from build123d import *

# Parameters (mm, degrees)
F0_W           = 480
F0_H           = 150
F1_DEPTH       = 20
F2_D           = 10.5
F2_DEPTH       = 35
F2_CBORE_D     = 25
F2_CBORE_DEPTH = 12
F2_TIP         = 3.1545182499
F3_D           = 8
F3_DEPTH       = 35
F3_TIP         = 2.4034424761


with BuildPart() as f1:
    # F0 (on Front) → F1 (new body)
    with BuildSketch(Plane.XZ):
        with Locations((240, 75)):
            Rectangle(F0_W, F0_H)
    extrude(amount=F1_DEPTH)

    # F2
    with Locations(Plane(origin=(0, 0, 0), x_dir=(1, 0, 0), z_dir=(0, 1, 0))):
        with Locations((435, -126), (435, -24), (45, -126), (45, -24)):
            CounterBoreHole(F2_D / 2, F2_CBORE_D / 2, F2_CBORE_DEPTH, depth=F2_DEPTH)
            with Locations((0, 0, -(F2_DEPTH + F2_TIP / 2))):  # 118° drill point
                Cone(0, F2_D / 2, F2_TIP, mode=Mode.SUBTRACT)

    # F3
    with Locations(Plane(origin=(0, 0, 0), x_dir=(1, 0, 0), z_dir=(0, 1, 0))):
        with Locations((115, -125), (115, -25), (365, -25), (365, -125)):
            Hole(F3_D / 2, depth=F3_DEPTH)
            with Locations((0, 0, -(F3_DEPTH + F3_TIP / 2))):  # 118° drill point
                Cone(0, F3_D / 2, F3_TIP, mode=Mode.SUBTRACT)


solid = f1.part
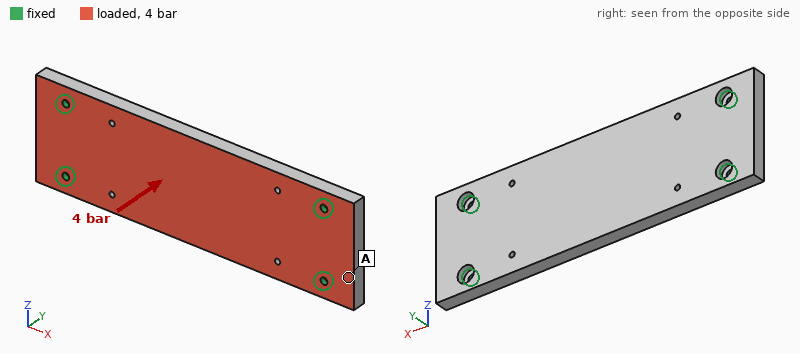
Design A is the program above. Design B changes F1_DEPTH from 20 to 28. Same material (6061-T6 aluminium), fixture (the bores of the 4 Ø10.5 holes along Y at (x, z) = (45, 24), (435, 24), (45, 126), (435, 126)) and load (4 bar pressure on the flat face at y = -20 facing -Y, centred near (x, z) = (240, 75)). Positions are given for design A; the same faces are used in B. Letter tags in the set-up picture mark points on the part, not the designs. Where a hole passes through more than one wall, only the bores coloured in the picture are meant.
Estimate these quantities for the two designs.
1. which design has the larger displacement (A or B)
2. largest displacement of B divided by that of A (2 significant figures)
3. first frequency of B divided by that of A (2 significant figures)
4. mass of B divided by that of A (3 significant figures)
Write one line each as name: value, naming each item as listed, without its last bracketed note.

which design has the larger displacement: A
largest displacement of B divided by that of A: 0.35
first frequency of B divided by that of A: 1.4
mass of B divided by that of A: 1.41
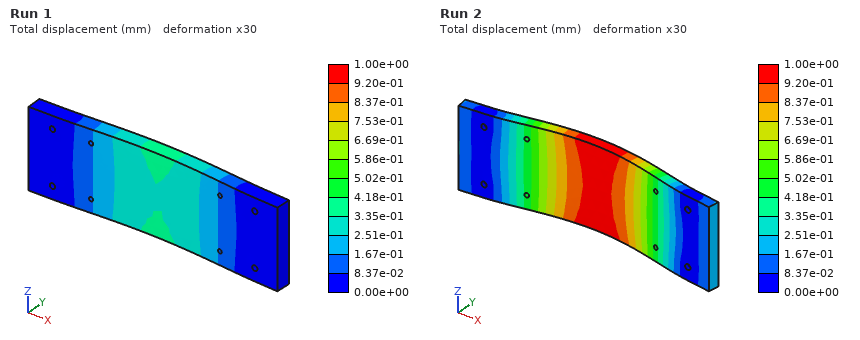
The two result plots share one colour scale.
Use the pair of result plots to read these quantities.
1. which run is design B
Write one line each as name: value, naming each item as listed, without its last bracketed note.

which run is design B: Run 1
